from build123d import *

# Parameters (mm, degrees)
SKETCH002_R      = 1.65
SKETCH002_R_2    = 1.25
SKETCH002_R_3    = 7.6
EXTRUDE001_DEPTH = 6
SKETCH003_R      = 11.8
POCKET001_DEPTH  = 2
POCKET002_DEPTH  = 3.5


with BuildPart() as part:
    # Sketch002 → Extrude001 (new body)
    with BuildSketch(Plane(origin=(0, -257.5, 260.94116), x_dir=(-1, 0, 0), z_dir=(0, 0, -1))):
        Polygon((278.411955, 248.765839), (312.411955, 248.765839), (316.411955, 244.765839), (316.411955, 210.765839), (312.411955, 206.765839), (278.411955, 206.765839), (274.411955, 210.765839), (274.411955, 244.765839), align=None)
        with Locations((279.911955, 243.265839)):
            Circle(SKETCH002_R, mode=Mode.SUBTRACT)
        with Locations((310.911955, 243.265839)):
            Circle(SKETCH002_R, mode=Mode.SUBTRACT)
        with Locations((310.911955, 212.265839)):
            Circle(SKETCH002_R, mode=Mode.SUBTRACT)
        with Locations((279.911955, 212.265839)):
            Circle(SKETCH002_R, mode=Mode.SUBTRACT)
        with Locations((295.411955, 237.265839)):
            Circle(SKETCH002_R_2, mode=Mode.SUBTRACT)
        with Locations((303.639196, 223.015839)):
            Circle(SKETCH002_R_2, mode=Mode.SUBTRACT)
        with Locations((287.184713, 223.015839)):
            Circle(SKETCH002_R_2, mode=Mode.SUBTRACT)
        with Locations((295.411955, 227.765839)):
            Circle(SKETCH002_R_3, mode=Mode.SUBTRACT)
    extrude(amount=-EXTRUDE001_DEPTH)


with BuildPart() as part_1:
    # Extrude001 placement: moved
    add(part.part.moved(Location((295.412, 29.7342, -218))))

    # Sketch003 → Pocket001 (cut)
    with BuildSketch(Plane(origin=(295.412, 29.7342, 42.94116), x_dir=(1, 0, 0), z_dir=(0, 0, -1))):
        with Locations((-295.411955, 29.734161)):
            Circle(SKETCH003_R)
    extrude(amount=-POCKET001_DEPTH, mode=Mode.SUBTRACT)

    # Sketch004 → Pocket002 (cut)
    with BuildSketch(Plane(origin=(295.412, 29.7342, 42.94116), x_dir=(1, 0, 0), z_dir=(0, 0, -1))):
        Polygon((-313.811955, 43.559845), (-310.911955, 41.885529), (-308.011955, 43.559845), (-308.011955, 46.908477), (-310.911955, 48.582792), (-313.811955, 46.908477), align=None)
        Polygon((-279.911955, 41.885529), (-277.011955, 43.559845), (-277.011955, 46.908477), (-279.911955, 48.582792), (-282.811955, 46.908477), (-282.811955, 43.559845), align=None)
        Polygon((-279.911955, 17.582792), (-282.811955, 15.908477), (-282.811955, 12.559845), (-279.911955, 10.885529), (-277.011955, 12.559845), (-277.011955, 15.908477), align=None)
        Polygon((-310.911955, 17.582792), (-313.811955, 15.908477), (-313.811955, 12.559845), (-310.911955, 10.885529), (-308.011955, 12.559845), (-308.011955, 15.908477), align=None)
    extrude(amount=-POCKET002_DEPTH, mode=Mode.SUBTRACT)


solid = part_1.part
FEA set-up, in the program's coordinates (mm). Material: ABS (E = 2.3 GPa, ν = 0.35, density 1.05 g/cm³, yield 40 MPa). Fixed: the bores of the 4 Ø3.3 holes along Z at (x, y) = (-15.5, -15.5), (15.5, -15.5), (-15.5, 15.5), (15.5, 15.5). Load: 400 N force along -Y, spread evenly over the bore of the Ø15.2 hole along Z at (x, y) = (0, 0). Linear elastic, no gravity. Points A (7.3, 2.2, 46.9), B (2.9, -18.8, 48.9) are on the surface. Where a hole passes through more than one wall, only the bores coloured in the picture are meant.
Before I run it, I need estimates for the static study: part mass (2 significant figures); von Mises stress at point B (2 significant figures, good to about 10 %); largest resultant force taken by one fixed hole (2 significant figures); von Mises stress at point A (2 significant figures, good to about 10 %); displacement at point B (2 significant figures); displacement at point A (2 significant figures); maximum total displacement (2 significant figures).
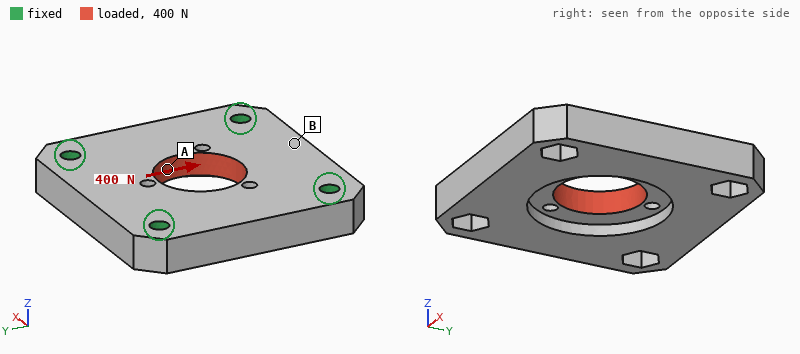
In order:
8.7 g
1.0 MPa
100 N
3.7 MPa
20 µm
21 µm
32 µm
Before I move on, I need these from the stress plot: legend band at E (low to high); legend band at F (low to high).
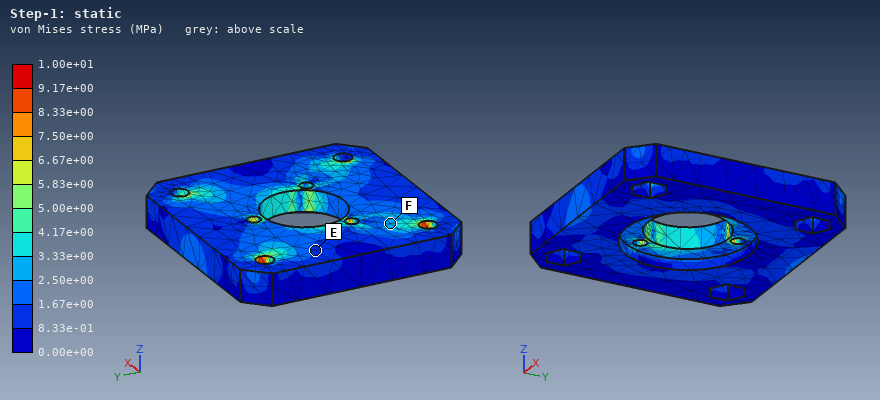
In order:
8.33e-01 to 1.67e+00 MPa
2.50e+00 to 3.33e+00 MPa
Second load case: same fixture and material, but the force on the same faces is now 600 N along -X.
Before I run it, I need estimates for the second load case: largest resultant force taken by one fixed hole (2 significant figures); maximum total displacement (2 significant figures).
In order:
160 N
44 µm
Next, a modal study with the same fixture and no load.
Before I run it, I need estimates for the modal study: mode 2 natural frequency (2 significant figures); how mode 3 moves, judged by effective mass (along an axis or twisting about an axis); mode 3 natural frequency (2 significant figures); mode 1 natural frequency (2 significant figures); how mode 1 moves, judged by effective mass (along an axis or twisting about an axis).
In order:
5800 Hz
twisting about X
6300 Hz
4800 Hz
along Z
